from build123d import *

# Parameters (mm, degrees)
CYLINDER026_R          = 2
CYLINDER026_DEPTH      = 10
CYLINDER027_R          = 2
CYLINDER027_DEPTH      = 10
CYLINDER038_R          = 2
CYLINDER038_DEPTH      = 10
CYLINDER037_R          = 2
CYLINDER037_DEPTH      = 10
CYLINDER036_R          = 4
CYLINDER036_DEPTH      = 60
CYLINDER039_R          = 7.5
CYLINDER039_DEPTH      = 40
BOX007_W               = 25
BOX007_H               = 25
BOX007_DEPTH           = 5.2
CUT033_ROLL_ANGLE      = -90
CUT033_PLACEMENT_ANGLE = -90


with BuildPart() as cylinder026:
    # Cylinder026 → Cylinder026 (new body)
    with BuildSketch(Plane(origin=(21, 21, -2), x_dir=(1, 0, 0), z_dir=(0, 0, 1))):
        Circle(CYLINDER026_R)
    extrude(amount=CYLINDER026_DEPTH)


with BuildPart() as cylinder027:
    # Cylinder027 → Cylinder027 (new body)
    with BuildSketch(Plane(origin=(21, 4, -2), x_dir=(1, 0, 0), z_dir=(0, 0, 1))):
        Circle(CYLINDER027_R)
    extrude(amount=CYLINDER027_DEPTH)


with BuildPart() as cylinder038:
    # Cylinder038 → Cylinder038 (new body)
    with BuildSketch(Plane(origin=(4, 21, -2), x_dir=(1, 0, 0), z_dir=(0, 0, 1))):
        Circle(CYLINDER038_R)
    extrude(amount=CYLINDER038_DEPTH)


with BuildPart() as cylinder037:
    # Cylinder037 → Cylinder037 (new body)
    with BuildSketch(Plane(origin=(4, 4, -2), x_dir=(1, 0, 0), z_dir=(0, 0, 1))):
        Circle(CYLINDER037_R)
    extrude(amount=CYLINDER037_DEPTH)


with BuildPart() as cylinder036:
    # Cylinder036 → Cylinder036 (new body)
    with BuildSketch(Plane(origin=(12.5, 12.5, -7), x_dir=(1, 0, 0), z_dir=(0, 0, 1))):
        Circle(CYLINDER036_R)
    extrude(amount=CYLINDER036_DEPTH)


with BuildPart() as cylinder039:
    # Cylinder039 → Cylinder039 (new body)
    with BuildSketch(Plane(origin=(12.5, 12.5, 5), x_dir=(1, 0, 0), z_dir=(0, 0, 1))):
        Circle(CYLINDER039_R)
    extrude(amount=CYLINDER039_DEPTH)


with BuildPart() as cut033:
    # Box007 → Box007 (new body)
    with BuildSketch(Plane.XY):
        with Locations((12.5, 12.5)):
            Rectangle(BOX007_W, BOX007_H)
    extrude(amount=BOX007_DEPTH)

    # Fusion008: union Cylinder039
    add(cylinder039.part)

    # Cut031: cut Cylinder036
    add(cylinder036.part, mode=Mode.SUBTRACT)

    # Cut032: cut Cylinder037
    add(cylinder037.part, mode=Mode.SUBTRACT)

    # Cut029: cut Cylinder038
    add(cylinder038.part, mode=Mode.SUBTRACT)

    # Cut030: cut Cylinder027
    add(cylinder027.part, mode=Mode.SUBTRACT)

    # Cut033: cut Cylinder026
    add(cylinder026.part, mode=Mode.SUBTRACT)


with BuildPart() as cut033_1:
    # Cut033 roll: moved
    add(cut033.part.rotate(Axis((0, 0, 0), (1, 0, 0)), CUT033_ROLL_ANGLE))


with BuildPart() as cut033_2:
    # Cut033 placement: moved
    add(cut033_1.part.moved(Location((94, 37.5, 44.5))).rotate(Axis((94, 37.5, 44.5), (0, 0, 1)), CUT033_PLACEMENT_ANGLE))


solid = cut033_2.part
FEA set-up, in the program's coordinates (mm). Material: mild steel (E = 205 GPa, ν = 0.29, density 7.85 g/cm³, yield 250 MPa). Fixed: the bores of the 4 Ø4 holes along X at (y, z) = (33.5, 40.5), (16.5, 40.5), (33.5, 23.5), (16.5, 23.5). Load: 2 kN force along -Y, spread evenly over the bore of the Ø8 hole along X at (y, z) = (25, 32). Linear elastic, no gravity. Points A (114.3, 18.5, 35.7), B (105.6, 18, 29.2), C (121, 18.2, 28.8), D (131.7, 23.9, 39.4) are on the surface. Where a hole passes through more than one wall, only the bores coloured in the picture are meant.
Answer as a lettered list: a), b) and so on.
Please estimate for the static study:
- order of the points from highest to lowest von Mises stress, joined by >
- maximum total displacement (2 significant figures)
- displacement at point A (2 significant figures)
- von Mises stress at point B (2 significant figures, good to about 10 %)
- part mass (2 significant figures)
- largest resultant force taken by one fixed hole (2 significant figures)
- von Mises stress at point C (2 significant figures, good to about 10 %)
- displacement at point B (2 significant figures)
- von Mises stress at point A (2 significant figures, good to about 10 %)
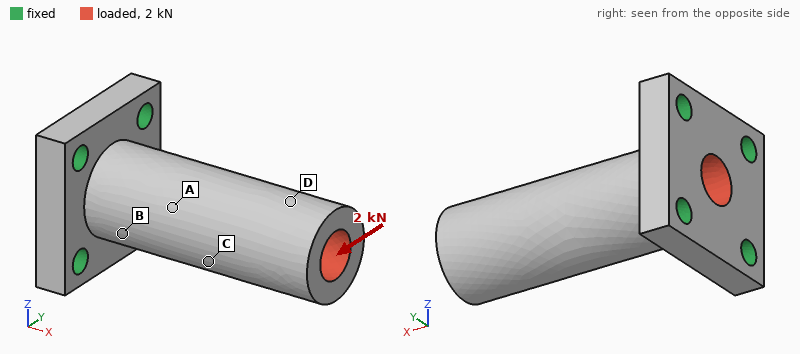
a) B > A > C > D
b) 57 µm
c) 20 µm
d) 73 MPa
e) 61 g
f) 1.5 kN
g) 22 MPa
h) 9.6 µm
i) 40 MPa
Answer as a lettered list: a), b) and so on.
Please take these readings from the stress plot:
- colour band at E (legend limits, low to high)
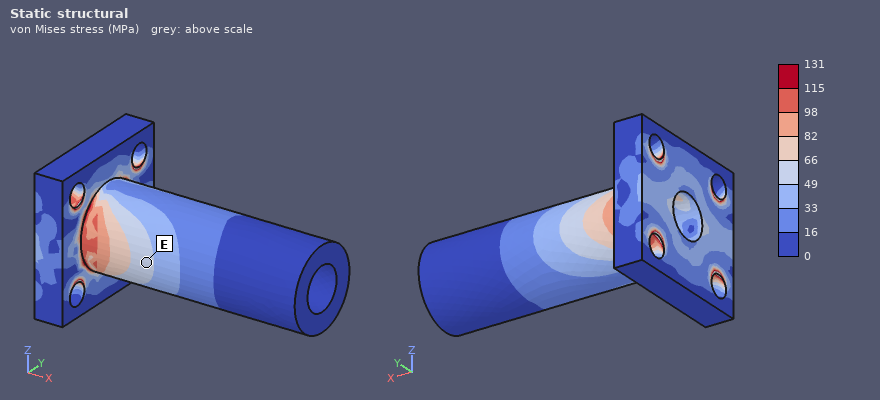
a) 49 to 66 MPa
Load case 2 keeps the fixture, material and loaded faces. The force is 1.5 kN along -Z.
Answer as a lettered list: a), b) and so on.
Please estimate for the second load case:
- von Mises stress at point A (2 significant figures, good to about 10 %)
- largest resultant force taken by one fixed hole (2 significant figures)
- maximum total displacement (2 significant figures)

a) 22 MPa
b) 1.1 kN
c) 42 µm
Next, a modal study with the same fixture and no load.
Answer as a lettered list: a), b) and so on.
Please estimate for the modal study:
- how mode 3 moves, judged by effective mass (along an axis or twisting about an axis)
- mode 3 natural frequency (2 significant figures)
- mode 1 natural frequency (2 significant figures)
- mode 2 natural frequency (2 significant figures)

a) twisting about X
b) 19 kHz
c) 5500 Hz
d) 5500 Hz
